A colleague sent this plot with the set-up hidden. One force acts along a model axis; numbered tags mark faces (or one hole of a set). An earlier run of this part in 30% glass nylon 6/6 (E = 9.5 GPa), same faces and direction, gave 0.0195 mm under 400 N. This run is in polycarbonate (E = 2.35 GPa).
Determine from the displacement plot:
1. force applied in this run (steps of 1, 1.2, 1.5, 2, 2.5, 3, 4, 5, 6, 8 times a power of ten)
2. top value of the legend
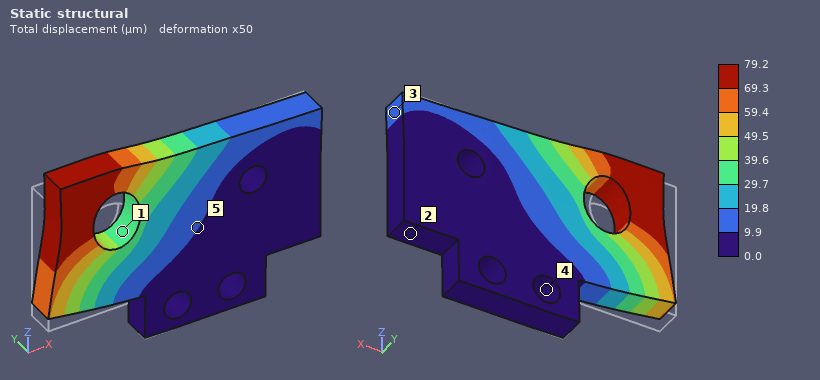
400 N
79.2 µm
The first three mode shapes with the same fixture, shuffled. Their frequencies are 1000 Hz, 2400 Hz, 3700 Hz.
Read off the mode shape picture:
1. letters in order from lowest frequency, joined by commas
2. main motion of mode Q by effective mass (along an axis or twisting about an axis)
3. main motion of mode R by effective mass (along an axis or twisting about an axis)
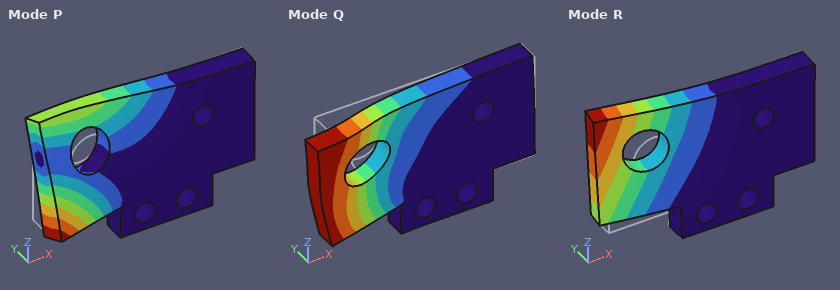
R, P, Q
along Z
along Y
